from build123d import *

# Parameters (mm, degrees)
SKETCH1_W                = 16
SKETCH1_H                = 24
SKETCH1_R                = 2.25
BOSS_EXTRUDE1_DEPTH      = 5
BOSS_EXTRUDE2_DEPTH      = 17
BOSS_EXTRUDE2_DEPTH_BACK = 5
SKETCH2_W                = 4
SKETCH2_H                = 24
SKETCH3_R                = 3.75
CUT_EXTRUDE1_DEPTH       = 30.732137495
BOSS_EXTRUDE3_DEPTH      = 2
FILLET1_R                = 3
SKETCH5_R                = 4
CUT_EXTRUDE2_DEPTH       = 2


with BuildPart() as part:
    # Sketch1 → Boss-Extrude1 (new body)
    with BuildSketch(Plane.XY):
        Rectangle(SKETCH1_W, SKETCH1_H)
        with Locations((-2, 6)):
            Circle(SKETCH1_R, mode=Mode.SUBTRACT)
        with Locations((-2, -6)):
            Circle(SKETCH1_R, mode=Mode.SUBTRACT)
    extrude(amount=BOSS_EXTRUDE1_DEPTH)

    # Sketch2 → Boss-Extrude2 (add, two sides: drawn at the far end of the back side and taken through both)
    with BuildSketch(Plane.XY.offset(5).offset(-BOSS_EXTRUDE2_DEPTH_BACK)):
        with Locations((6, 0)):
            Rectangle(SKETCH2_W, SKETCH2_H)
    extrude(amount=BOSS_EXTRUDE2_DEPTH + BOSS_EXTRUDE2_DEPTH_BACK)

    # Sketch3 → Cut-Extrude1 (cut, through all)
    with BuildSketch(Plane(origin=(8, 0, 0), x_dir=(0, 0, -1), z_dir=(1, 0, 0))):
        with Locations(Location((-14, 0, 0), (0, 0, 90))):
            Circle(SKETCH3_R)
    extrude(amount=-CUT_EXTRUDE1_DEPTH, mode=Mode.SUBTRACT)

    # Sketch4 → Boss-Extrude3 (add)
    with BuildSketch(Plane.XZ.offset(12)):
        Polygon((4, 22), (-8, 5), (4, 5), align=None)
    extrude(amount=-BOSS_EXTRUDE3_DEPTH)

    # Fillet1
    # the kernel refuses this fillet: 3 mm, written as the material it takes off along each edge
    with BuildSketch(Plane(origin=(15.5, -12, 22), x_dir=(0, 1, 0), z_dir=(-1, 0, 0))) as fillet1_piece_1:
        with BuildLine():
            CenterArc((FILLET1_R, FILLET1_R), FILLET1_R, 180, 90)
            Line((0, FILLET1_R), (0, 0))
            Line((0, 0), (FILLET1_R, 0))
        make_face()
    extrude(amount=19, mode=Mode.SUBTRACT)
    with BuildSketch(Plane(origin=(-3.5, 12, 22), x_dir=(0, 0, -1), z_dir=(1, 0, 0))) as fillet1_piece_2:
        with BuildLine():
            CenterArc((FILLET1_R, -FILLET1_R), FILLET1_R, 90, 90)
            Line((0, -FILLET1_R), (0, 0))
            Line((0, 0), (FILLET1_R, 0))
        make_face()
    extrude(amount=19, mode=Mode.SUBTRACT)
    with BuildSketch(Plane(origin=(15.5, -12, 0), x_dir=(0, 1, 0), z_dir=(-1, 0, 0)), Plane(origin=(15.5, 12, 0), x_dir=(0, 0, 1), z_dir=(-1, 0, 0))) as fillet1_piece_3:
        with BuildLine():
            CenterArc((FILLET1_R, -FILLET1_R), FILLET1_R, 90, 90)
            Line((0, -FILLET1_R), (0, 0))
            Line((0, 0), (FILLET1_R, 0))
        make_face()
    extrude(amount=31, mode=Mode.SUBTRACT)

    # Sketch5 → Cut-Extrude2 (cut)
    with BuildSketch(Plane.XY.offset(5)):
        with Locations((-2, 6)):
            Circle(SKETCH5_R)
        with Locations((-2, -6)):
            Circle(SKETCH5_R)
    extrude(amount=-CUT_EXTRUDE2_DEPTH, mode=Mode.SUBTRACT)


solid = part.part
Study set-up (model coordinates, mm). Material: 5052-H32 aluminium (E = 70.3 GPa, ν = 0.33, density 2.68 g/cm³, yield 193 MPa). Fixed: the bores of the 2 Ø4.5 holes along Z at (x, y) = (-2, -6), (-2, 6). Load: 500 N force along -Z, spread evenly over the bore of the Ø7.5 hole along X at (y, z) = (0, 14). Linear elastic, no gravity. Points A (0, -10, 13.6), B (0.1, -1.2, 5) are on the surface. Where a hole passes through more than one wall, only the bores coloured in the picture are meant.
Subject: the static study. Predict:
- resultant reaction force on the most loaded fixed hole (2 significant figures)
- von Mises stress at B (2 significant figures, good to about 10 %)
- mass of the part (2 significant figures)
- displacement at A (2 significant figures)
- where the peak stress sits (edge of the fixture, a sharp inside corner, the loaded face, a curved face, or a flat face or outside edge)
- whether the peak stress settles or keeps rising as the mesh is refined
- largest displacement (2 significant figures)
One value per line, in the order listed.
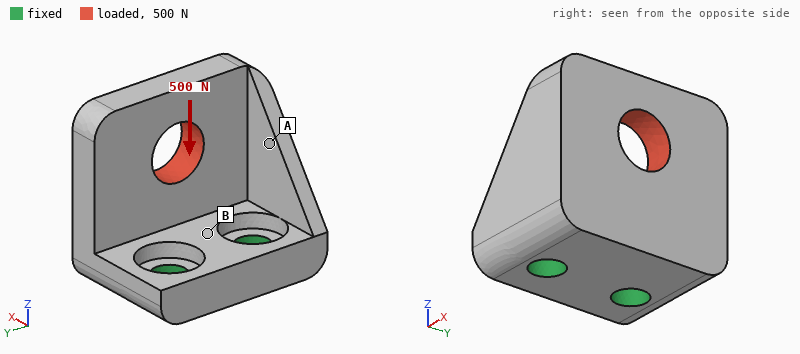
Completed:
250 N
28 MPa
8.6 g
13 µm
edge of the fixture
keeps rising
30 µm
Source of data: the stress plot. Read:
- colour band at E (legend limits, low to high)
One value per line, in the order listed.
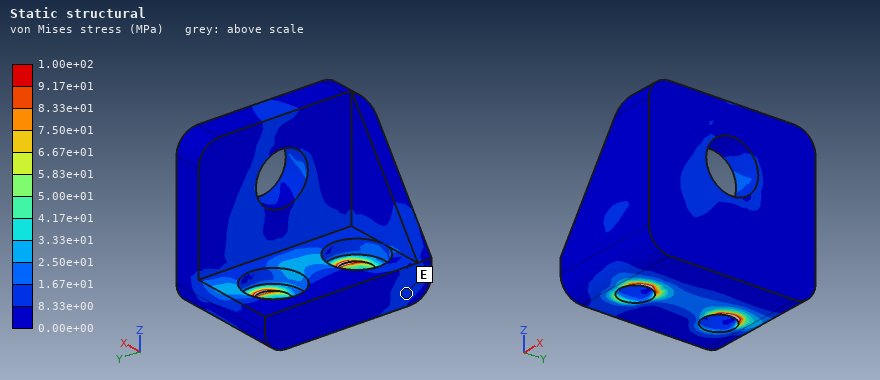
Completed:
8.33e+00 to 1.67e+01 MPa
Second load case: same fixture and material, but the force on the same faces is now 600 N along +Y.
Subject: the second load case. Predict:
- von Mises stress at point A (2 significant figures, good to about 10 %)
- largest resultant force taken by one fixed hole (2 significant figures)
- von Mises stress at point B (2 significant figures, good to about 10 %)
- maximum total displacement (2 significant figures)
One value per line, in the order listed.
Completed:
13 MPa
660 N
27 MPa
36 µm
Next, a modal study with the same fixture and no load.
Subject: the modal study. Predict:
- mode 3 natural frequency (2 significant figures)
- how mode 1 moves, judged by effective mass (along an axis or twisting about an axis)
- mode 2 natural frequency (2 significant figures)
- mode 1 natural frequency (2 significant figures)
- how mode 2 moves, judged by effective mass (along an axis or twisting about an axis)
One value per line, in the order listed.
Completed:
18 kHz
along X
11 kHz
7100 Hz
along Y
